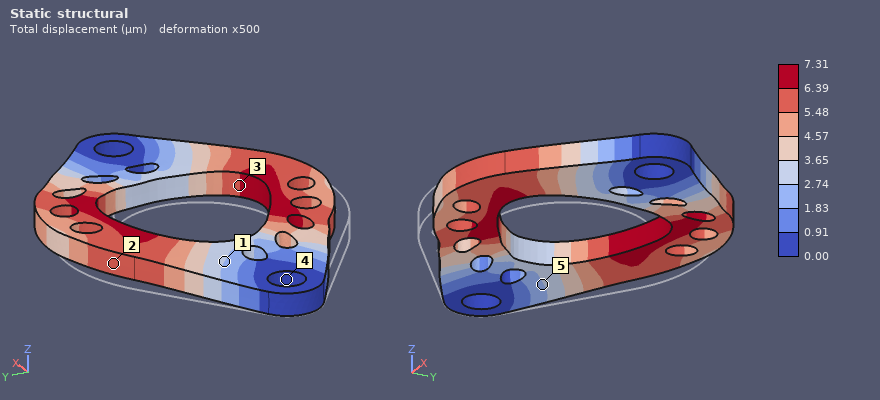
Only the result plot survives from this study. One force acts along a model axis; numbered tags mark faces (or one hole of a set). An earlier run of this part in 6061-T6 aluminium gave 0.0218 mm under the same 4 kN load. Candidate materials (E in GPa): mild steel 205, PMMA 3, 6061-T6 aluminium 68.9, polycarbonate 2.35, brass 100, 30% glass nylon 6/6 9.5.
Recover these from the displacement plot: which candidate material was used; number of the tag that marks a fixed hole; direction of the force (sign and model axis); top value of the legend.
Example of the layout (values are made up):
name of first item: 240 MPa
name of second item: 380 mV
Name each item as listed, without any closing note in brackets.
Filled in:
which candidate material was used: mild steel
number of the tag that marks a fixed hole: 4
direction of the force: +X
top value of the legend: 7.31 µm
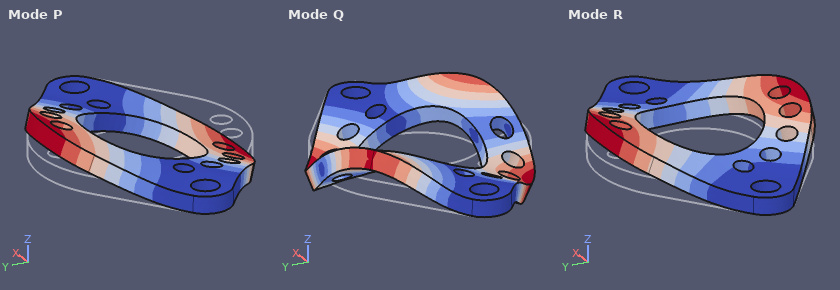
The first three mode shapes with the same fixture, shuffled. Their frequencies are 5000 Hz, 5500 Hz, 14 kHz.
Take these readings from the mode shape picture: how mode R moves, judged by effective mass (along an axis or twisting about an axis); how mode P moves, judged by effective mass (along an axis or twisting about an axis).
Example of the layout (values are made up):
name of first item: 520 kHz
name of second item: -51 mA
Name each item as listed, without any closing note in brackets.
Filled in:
how mode R moves, judged by effective mass: along Z
how mode P moves, judged by effective mass: twisting about X
